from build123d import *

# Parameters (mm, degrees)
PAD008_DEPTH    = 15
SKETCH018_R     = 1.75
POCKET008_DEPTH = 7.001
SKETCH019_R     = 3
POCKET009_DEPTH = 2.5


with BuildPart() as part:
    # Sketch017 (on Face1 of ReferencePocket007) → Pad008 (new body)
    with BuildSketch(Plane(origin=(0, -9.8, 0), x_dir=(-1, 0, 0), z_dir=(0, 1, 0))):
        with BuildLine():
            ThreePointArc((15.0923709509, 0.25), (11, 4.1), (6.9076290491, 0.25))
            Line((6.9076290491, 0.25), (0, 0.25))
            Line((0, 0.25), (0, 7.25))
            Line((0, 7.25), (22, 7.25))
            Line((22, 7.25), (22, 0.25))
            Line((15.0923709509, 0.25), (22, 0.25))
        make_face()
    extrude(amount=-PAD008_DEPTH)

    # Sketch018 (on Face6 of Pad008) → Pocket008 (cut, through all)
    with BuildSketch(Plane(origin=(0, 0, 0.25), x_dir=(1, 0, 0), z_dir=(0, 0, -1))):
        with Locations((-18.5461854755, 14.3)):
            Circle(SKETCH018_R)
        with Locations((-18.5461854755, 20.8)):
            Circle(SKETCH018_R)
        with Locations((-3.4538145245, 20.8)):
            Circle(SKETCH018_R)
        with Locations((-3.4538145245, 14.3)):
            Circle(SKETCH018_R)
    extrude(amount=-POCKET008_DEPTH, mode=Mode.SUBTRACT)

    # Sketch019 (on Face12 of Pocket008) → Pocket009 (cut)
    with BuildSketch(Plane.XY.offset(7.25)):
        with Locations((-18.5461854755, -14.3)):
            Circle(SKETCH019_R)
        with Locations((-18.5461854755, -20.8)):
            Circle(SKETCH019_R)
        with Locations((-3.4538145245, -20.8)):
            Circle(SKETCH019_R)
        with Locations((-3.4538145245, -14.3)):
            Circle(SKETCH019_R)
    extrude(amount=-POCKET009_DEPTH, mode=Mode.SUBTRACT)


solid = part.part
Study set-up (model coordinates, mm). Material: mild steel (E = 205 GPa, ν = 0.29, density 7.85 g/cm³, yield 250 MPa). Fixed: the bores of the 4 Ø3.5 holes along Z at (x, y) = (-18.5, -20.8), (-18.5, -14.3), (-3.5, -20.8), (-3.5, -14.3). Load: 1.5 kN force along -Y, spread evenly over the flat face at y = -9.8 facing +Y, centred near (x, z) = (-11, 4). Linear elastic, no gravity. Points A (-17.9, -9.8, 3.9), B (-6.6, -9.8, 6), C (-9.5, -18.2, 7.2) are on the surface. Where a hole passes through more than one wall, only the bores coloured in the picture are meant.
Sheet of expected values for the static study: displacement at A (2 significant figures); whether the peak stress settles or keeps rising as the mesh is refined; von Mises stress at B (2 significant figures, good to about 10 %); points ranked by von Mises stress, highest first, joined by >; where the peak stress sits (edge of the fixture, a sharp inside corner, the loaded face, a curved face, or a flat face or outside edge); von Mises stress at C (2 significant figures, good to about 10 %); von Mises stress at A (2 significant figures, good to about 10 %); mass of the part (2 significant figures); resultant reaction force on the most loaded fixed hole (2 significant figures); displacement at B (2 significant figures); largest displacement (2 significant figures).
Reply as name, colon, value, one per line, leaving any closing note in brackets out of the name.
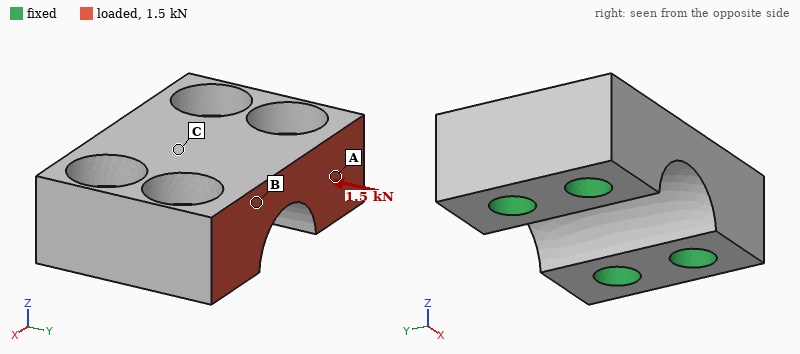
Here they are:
displacement at A: 0.52 µm
whether the peak stress settles or keeps rising as the mesh is refined: keeps rising
von Mises stress at B: 18 MPa
points ranked by von Mises stress, highest first, joined by >: A > B > C
where the peak stress sits: edge of the fixture
von Mises stress at C: 7.5 MPa
von Mises stress at A: 29 MPa
mass of the part: 12 g
resultant reaction force on the most loaded fixed hole: 600 N
displacement at B: 0.98 µm
largest displacement: 1.5 µm
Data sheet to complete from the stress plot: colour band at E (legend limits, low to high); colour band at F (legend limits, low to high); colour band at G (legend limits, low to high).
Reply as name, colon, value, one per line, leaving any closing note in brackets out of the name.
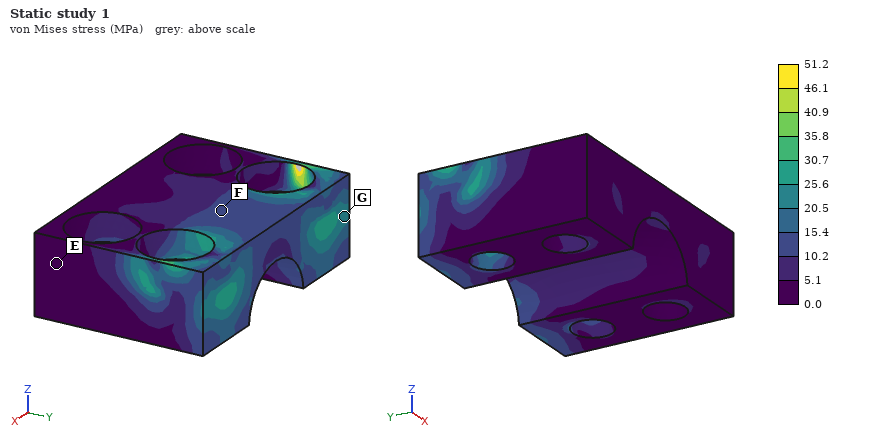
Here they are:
colour band at E: 0.0 to 5.1 MPa
colour band at F: 10.2 to 15.4 MPa
colour band at G: 20.5 to 25.6 MPa
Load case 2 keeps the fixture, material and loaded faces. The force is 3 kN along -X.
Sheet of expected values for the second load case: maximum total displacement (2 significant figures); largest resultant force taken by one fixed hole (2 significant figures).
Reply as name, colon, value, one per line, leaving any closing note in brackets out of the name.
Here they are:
maximum total displacement: 3.8 µm
largest resultant force taken by one fixed hole: 1.5 kN
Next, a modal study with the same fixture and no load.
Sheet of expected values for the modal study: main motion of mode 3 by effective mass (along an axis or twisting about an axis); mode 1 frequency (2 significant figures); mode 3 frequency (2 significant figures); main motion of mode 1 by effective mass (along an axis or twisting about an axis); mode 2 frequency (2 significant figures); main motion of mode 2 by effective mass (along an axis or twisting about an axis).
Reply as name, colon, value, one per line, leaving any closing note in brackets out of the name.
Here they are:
main motion of mode 3 by effective mass: along X
mode 1 frequency: 78 kHz
mode 3 frequency: 110 kHz
main motion of mode 1 by effective mass: along Y
mode 2 frequency: 95 kHz
main motion of mode 2 by effective mass: along Z
